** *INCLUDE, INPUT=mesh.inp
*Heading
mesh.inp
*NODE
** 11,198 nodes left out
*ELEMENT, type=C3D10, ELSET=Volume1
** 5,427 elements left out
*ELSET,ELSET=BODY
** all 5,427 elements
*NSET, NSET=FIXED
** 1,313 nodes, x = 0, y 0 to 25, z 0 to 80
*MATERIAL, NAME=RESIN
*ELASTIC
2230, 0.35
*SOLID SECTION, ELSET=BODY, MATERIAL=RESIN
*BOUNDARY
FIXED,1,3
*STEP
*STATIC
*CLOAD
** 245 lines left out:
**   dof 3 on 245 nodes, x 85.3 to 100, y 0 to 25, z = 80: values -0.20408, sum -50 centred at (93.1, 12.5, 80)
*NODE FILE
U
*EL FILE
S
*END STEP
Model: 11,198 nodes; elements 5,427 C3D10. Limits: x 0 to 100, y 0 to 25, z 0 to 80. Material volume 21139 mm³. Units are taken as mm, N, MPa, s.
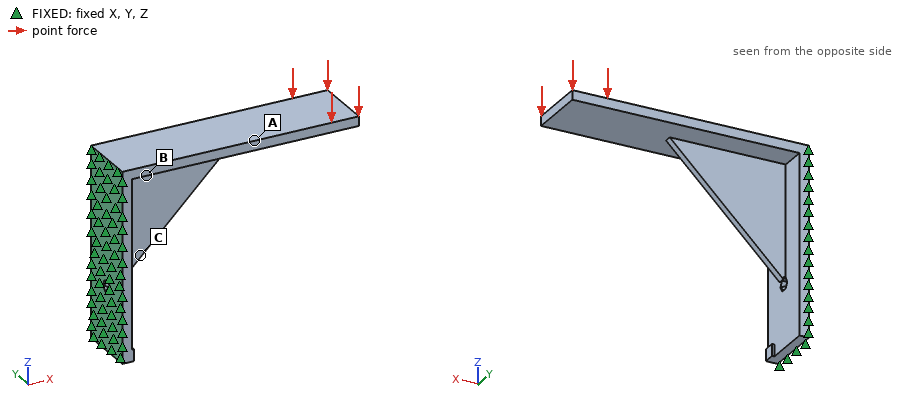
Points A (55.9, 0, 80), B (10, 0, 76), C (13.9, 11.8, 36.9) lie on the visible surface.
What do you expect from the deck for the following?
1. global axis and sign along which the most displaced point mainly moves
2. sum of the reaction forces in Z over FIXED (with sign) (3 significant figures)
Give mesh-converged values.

-Z
50.0 N
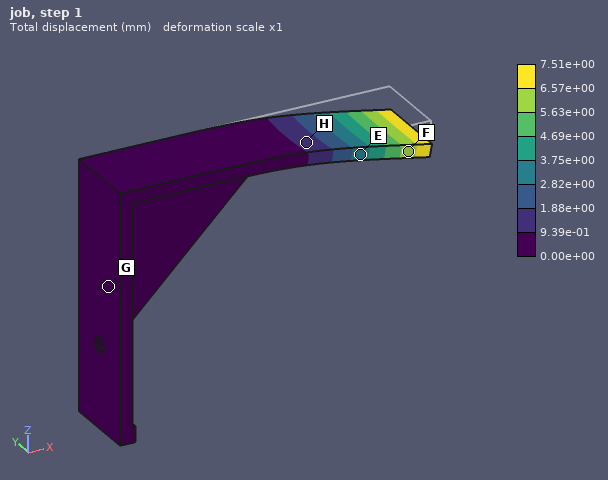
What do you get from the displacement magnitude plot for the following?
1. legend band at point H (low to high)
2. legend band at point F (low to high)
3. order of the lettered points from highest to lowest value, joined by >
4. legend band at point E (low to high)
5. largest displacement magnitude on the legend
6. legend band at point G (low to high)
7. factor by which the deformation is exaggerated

9.39e-01 to 1.88e+00 mm
5.63e+00 to 6.57e+00 mm
F > E > H > G
2.82e+00 to 3.75e+00 mm
7.51e+00 mm
0.00e+00 to 9.39e-01 mm
1
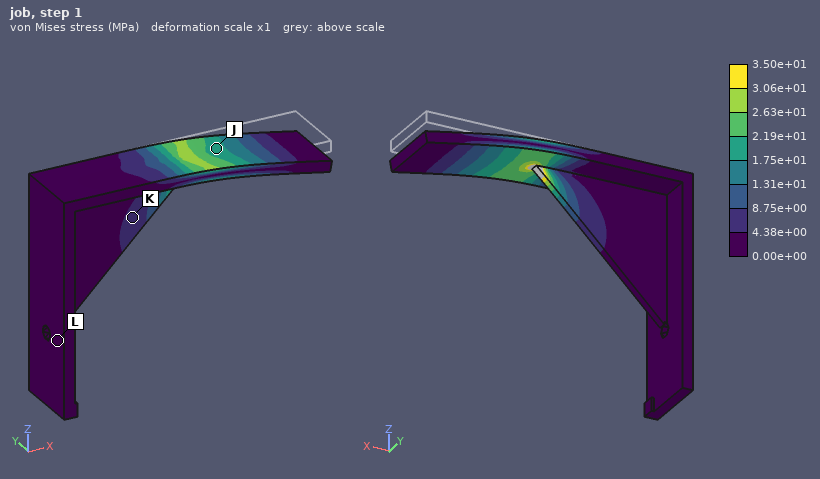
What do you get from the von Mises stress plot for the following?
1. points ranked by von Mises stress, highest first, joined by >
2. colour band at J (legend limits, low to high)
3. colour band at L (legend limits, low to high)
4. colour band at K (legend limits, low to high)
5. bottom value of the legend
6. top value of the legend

J > K > L
1.75e+01 to 2.19e+01 MPa
0.00e+00 to 4.38e+00 MPa
4.38e+00 to 8.75e+00 MPa
0.00e+00 MPa
3.50e+01 MPa
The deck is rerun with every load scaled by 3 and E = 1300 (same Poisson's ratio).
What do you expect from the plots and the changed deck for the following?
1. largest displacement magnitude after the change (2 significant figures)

39 mm
